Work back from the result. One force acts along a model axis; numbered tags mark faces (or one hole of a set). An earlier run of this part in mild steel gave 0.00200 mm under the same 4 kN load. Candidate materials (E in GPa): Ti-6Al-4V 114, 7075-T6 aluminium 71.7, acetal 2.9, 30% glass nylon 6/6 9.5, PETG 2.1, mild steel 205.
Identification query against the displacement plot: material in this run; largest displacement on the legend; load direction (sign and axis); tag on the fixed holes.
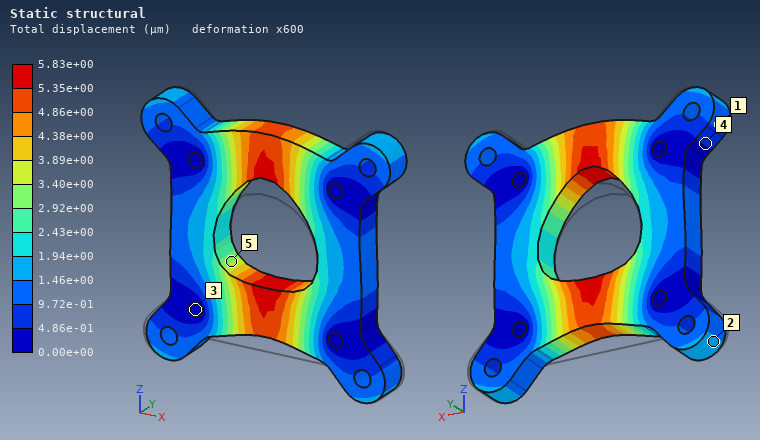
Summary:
7075-T6 aluminium
5.83e+00 µm
+Z
3
